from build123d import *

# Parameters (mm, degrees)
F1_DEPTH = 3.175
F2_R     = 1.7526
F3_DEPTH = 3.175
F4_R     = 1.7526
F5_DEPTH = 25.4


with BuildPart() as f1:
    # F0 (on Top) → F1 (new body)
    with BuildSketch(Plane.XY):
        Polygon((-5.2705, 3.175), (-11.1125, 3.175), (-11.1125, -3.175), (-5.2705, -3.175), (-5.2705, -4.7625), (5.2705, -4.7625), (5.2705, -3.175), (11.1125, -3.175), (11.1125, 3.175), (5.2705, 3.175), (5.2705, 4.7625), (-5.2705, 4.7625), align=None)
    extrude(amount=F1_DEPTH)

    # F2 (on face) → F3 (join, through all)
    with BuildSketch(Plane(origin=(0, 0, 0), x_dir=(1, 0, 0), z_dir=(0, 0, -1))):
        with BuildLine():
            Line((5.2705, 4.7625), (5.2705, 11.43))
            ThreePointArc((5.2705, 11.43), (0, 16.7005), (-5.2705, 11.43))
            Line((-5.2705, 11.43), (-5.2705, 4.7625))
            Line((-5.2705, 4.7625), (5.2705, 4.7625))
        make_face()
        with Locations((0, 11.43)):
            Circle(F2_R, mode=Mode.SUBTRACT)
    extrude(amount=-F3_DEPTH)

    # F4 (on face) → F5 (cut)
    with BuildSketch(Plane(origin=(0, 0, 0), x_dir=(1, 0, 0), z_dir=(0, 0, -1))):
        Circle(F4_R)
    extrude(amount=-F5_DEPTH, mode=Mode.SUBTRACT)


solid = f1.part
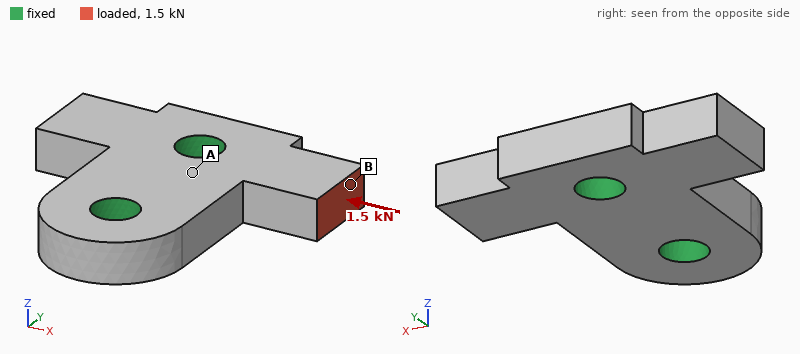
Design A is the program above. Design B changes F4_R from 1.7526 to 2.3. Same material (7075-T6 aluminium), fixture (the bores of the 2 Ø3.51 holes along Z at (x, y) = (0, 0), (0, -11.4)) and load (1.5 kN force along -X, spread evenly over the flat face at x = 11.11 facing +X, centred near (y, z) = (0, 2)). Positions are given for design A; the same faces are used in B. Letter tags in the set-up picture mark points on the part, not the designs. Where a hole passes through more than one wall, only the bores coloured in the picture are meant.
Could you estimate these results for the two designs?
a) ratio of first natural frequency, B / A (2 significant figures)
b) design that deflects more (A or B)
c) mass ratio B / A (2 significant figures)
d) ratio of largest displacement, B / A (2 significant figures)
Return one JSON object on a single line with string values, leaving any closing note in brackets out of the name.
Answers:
{"ratio of first natural frequency, B / A": "1.1", "design that deflects more": "A", "mass ratio B / A": "0.97", "ratio of largest displacement, B / A": "0.90"}
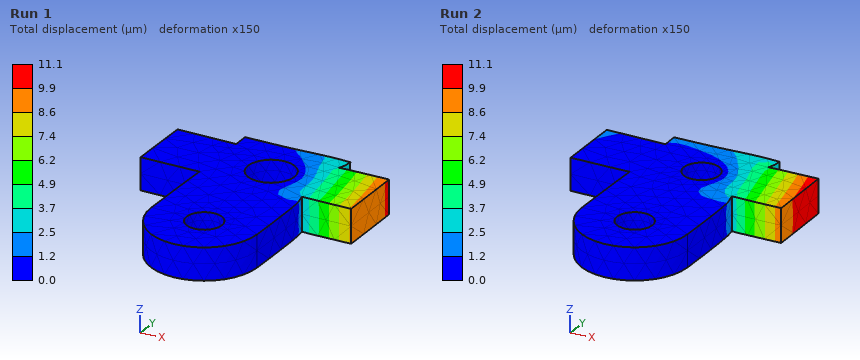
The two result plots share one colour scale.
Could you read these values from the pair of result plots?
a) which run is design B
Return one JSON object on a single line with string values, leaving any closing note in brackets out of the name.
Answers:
{"which run is design B": "Run 1"}
